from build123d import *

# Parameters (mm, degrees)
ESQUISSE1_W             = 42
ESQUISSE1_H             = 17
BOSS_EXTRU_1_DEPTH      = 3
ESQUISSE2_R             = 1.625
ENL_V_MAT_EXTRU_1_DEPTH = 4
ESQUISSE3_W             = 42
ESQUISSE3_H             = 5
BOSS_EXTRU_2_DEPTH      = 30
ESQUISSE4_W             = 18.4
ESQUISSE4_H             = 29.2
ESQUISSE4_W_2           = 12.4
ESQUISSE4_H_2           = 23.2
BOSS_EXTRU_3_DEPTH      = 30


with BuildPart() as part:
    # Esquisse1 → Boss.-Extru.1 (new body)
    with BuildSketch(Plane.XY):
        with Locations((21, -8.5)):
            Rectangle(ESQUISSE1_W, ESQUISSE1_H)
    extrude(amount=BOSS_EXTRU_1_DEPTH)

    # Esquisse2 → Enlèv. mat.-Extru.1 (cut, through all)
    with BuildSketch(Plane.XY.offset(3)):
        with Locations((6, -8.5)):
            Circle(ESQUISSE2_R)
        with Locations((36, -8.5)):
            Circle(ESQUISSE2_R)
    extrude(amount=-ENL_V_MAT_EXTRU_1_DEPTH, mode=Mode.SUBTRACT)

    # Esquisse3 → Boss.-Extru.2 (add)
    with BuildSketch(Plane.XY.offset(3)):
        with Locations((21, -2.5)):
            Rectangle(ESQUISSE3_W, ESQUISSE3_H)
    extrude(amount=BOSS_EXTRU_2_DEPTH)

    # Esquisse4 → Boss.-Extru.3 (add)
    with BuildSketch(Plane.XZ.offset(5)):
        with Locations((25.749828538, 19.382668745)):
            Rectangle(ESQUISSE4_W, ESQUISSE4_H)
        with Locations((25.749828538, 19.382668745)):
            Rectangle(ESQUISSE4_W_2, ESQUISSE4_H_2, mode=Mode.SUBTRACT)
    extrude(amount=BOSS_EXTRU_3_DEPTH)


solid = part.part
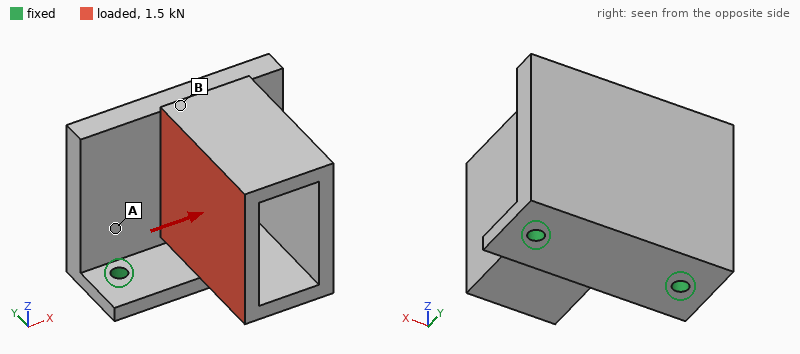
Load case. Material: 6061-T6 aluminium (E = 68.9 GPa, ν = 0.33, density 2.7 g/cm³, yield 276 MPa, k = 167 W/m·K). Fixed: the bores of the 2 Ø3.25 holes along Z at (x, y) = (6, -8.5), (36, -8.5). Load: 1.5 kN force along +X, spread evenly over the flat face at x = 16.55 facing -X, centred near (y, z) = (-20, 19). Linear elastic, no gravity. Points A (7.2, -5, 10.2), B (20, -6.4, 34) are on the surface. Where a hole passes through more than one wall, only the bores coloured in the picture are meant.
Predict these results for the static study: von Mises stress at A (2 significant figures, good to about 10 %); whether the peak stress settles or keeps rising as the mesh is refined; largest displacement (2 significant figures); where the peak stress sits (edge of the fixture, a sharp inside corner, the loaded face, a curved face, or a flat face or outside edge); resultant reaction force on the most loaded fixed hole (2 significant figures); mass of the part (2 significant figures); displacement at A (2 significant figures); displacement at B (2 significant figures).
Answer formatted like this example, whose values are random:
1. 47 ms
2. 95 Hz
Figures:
1. 62 MPa
2. keeps rising
3. 0.22 mm
4. edge of the fixture
5. 1.4 kN
6. 43 g
7. 0.039 mm
8. 0.073 mm
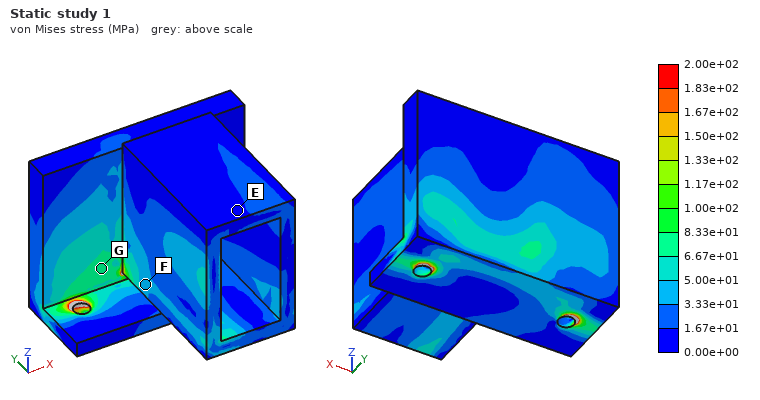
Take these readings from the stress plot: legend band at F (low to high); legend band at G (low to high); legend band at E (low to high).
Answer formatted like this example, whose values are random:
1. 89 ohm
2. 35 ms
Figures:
1. 3.33e+01 to 5.00e+01 MPa
2. 6.67e+01 to 8.33e+01 MPa
3. 0.00e+00 to 1.67e+01 MPa
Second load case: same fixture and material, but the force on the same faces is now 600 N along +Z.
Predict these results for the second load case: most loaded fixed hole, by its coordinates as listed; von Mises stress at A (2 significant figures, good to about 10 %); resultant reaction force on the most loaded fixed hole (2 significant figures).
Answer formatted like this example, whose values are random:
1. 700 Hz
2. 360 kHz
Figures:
1. (6, -8.5)
2. 38 MPa
3. 390 N
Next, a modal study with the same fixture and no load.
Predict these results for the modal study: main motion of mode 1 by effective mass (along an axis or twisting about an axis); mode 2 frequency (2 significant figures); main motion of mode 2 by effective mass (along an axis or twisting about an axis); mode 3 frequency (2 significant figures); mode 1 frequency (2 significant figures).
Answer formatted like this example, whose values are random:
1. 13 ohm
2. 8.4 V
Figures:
1. along Y
2. 3400 Hz
3. along X
4. 7100 Hz
5. 1100 Hz
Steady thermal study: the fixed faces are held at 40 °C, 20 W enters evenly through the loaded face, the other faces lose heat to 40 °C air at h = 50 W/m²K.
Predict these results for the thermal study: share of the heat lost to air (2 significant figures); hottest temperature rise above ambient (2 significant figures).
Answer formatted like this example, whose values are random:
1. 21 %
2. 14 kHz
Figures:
1. 24 %
2. 21 K
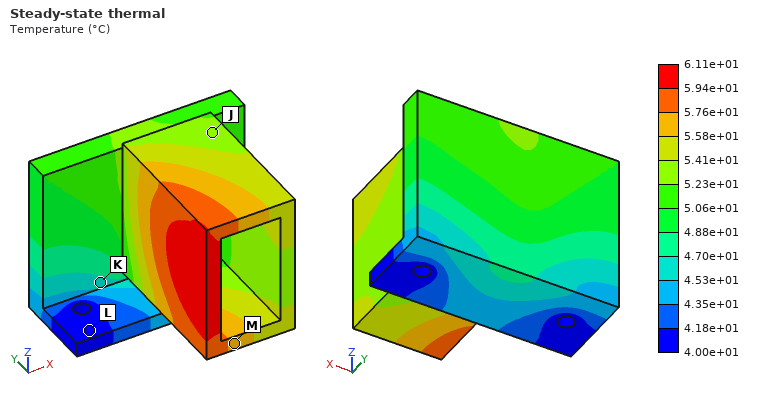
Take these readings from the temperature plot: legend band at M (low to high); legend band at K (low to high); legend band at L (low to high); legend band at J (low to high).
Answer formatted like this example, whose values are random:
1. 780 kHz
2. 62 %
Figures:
1. 5.58e+01 to 5.76e+01 °C
2. 4.53e+01 to 4.70e+01 °C
3. 4.00e+01 to 4.18e+01 °C
4. 5.23e+01 to 5.41e+01 °C
